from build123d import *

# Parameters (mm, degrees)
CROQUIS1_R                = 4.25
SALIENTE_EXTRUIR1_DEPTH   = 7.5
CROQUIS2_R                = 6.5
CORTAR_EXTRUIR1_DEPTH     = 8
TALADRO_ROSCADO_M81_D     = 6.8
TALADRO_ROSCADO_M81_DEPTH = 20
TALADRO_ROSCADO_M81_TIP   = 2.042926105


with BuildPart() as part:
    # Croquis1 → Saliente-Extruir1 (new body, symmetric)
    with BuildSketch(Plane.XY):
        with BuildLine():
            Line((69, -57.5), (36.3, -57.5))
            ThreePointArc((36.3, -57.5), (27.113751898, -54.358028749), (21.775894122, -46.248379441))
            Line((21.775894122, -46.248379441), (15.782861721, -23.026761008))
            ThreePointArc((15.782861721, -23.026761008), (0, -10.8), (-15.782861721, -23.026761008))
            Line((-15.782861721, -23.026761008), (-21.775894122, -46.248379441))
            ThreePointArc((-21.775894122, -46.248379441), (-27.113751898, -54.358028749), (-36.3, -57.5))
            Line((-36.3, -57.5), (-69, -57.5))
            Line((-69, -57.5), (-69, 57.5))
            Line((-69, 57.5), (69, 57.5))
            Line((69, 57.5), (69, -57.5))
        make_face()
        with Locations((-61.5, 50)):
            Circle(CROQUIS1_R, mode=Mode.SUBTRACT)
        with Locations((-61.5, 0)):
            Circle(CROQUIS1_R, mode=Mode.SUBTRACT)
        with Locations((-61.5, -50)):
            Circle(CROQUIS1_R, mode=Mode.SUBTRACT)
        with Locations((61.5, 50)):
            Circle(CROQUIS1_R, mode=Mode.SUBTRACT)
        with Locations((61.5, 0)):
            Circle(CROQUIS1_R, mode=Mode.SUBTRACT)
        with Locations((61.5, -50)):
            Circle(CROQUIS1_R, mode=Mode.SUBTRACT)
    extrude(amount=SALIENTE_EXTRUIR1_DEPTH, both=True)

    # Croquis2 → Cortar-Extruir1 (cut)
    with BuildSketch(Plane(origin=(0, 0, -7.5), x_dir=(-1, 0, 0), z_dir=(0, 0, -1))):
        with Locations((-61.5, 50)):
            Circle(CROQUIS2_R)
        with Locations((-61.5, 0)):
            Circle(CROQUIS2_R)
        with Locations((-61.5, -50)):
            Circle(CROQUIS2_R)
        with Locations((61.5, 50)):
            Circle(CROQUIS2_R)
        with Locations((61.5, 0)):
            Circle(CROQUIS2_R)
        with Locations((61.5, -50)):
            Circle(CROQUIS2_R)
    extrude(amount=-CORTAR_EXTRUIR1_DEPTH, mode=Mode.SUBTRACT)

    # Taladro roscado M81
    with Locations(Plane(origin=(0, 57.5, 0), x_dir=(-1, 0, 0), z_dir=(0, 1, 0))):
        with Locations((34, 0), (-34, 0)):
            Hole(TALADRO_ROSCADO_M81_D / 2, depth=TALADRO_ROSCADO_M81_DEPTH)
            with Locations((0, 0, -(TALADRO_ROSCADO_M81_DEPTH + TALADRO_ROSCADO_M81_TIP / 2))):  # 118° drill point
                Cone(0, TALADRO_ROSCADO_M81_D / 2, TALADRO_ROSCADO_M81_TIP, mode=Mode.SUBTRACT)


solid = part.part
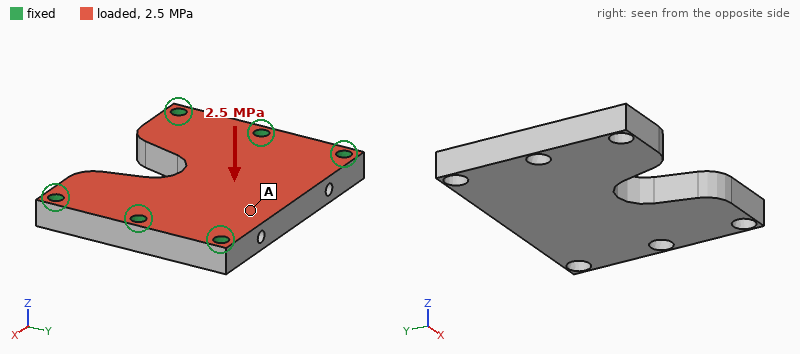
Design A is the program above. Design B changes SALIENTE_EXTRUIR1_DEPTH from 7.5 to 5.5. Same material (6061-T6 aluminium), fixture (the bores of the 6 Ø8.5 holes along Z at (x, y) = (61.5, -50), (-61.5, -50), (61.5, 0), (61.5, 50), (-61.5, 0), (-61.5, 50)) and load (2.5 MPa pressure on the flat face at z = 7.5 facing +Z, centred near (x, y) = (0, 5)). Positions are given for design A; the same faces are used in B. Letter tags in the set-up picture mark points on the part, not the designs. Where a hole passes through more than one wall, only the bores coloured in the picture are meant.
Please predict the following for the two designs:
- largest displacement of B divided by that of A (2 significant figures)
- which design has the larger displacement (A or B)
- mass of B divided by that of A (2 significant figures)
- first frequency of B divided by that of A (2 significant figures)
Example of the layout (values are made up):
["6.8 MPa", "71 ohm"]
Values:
["2.2", "B", "0.73", "0.80"]
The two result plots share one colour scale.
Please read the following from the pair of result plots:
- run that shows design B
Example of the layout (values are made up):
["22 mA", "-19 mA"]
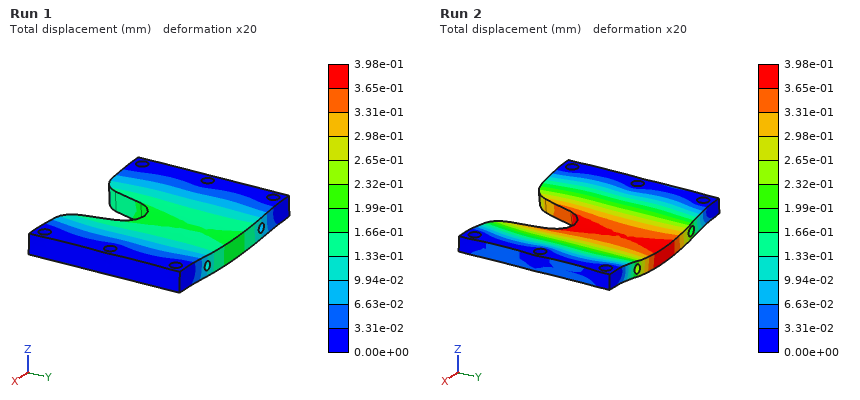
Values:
["Run 2"]
